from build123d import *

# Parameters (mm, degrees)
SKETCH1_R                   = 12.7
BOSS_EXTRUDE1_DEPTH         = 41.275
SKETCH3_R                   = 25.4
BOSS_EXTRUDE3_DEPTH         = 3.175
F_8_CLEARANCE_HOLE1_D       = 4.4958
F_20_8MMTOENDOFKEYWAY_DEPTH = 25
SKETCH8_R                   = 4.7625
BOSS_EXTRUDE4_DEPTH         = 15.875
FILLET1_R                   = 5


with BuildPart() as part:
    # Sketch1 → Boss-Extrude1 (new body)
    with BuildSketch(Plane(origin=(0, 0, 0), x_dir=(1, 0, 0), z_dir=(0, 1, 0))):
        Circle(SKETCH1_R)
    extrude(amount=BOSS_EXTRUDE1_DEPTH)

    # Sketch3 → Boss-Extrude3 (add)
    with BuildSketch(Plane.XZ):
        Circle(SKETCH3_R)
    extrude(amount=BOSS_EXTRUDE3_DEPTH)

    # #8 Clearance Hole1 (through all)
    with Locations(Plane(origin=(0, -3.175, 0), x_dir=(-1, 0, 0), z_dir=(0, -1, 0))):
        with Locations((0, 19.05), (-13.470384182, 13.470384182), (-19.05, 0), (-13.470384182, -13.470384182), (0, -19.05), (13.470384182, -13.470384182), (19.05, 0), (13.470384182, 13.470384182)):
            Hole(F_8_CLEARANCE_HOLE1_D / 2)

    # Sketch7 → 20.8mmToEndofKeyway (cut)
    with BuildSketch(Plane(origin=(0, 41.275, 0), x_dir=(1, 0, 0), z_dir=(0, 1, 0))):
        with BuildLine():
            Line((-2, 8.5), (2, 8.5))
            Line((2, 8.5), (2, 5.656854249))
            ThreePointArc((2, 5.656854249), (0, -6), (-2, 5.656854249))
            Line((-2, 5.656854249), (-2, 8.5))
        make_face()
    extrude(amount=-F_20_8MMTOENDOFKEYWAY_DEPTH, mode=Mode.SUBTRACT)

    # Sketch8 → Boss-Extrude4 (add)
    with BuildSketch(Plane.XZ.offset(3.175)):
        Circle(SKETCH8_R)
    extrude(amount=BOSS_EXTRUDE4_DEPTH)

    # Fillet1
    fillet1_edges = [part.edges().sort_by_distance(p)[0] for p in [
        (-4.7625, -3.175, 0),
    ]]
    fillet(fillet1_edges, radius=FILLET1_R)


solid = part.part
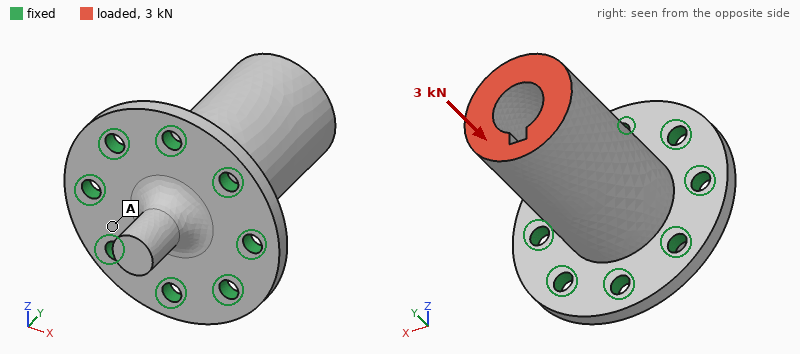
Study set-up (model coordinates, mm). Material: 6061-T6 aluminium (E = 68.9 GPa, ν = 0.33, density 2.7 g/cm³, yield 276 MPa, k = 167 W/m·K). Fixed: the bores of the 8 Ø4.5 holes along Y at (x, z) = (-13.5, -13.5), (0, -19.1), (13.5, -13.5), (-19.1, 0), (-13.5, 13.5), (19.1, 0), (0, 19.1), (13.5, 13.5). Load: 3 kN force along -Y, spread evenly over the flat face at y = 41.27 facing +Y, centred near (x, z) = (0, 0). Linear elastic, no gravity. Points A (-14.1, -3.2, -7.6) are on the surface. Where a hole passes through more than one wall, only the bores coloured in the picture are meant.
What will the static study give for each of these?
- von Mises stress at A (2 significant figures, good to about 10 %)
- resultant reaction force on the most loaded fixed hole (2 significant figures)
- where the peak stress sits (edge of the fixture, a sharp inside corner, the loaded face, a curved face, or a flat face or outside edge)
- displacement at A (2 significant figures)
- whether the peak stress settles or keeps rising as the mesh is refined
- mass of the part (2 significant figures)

16 MPa
420 N
edge of the fixture
3.2 µm
keeps rising
68 g
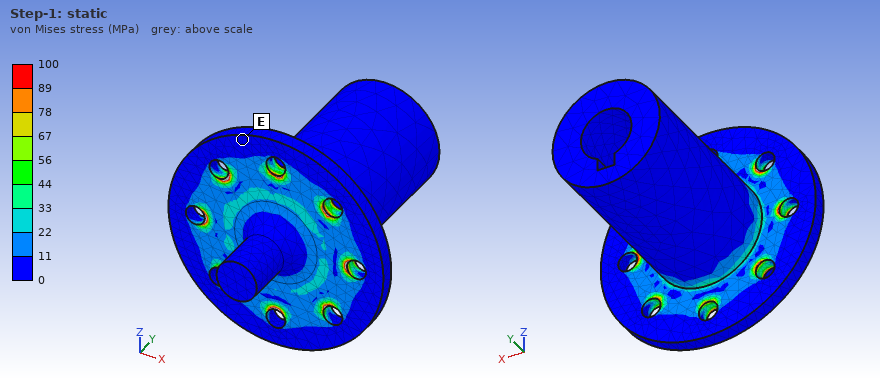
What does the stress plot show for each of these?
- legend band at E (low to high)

0 to 11 MPa
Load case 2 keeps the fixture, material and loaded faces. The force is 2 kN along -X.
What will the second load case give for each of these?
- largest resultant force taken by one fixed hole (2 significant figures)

1.5 kN
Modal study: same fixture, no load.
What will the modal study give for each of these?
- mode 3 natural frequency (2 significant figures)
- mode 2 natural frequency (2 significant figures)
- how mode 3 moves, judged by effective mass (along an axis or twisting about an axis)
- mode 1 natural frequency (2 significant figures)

12 kHz
5300 Hz
along Y
5200 Hz
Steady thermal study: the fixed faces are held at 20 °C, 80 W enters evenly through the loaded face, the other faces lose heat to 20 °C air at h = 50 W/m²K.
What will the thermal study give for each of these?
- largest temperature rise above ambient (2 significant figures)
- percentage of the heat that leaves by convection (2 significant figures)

57 K
11 %
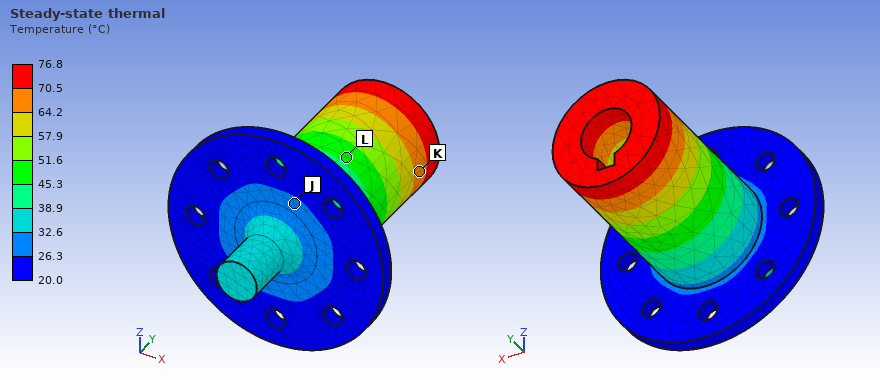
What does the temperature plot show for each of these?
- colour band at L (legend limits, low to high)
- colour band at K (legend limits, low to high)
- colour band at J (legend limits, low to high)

45.3 to 51.6 °C
64.2 to 70.5 °C
26.3 to 32.6 °C
